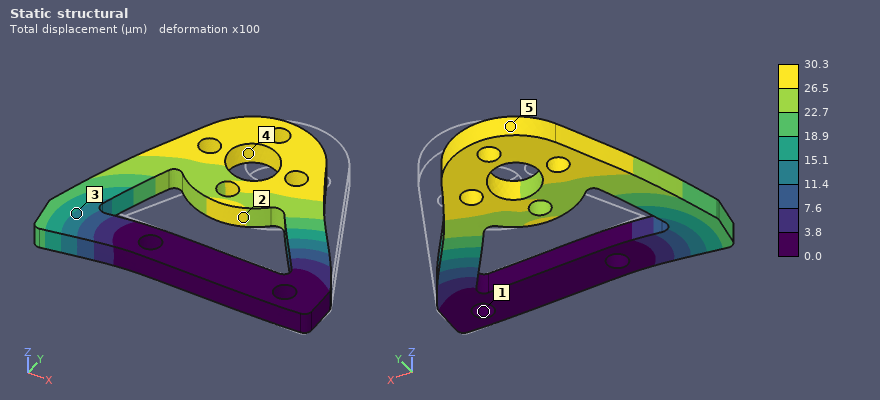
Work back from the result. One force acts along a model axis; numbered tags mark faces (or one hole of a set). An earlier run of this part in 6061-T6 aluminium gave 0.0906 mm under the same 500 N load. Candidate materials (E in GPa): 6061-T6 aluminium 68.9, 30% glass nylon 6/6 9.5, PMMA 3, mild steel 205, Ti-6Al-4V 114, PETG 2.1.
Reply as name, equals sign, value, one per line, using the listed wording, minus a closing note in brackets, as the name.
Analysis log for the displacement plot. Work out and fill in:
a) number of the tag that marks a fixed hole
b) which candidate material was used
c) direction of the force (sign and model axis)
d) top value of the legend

number of the tag that marks a fixed hole = 1
which candidate material was used = mild steel
direction of the force = -X
top value of the legend = 30.3 µm
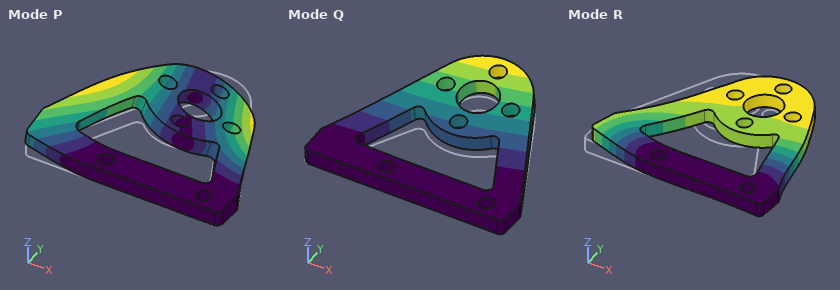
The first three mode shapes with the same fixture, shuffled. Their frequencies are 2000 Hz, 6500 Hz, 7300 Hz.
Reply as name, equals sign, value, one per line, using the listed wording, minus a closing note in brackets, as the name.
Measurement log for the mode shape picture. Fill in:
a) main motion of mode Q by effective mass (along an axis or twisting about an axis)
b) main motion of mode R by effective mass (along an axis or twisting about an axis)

main motion of mode Q by effective mass = along Z
main motion of mode R by effective mass = along X
